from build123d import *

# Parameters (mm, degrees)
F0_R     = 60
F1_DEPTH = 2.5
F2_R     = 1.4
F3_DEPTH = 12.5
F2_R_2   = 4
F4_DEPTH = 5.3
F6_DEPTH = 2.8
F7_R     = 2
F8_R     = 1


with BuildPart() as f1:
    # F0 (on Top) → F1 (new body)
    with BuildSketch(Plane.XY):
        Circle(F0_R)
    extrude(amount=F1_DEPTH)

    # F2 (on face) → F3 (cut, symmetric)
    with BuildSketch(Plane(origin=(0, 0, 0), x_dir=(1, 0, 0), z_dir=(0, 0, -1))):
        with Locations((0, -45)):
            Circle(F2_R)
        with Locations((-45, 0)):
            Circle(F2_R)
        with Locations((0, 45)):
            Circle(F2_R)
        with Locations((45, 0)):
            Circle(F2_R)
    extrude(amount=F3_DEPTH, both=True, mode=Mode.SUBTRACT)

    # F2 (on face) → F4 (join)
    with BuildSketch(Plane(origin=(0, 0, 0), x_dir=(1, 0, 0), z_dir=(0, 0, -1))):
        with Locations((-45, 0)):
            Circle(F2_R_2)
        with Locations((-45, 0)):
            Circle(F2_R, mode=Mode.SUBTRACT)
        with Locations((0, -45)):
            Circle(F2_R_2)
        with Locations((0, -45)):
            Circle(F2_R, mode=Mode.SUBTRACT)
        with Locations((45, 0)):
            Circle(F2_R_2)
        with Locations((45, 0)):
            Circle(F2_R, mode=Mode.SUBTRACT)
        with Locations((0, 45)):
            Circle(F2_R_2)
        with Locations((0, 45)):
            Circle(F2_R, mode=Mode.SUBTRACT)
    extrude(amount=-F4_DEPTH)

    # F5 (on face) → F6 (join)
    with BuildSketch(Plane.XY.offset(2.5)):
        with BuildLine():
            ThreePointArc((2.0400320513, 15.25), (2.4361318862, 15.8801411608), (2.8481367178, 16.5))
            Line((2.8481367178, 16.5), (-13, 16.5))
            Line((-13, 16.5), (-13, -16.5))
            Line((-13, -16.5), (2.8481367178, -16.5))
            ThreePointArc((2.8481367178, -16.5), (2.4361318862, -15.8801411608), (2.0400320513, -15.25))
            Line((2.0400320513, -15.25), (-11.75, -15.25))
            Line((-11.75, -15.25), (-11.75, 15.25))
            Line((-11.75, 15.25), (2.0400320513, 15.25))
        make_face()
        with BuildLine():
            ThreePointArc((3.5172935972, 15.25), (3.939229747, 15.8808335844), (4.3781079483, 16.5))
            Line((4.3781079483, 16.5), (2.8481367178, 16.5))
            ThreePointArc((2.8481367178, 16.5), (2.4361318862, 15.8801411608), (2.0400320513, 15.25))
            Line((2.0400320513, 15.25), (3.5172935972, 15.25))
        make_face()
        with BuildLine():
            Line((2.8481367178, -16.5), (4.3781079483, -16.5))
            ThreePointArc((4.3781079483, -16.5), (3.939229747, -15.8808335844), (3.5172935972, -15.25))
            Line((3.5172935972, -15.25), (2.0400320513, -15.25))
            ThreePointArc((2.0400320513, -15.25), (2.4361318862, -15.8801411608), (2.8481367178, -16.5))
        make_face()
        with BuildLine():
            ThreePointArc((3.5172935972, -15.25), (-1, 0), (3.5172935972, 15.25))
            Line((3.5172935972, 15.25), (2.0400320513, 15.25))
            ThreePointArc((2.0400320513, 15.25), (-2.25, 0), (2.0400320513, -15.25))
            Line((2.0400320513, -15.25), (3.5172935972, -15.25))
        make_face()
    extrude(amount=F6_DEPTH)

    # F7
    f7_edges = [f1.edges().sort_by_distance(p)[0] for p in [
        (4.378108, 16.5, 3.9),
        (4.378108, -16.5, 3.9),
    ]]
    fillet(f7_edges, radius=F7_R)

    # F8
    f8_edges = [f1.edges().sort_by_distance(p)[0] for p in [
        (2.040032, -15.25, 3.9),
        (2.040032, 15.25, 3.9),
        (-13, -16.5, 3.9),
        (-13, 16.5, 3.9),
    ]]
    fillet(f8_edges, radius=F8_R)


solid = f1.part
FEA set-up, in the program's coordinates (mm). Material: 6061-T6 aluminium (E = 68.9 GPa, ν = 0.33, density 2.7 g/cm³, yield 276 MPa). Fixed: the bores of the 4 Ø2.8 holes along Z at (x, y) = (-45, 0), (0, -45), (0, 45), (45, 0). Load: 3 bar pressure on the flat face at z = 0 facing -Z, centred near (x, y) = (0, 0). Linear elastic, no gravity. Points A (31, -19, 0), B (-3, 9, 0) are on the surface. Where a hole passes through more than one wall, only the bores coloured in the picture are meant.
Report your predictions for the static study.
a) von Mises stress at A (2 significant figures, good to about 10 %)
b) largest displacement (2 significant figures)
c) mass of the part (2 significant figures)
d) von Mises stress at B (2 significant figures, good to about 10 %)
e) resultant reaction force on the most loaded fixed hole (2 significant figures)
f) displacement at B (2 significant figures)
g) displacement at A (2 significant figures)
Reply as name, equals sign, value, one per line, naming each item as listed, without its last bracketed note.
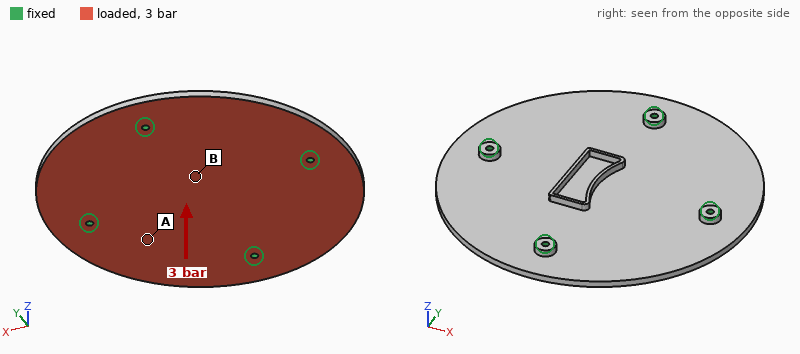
von Mises stress at A = 58 MPa
largest displacement = 0.32 mm
mass of the part = 78 g
von Mises stress at B = 31 MPa
resultant reaction force on the most loaded fixed hole = 860 N
displacement at B = 0.22 mm
displacement at A = 0.16 mm
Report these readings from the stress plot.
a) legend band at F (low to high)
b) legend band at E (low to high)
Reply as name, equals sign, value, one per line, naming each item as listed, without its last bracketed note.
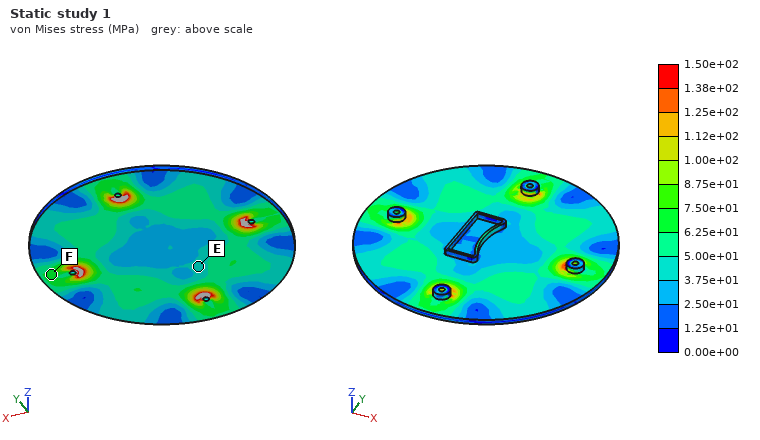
legend band at F = 6.25e+01 to 7.50e+01 MPa
legend band at E = 3.75e+01 to 5.00e+01 MPa
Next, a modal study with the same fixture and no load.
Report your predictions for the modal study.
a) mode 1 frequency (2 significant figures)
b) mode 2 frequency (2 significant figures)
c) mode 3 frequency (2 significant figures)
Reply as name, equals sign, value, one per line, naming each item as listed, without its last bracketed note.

mode 1 frequency = 2100 Hz
mode 2 frequency = 2200 Hz
mode 3 frequency = 2200 Hz
